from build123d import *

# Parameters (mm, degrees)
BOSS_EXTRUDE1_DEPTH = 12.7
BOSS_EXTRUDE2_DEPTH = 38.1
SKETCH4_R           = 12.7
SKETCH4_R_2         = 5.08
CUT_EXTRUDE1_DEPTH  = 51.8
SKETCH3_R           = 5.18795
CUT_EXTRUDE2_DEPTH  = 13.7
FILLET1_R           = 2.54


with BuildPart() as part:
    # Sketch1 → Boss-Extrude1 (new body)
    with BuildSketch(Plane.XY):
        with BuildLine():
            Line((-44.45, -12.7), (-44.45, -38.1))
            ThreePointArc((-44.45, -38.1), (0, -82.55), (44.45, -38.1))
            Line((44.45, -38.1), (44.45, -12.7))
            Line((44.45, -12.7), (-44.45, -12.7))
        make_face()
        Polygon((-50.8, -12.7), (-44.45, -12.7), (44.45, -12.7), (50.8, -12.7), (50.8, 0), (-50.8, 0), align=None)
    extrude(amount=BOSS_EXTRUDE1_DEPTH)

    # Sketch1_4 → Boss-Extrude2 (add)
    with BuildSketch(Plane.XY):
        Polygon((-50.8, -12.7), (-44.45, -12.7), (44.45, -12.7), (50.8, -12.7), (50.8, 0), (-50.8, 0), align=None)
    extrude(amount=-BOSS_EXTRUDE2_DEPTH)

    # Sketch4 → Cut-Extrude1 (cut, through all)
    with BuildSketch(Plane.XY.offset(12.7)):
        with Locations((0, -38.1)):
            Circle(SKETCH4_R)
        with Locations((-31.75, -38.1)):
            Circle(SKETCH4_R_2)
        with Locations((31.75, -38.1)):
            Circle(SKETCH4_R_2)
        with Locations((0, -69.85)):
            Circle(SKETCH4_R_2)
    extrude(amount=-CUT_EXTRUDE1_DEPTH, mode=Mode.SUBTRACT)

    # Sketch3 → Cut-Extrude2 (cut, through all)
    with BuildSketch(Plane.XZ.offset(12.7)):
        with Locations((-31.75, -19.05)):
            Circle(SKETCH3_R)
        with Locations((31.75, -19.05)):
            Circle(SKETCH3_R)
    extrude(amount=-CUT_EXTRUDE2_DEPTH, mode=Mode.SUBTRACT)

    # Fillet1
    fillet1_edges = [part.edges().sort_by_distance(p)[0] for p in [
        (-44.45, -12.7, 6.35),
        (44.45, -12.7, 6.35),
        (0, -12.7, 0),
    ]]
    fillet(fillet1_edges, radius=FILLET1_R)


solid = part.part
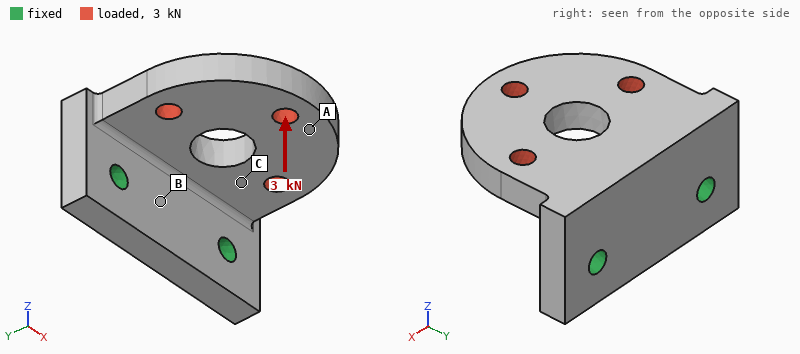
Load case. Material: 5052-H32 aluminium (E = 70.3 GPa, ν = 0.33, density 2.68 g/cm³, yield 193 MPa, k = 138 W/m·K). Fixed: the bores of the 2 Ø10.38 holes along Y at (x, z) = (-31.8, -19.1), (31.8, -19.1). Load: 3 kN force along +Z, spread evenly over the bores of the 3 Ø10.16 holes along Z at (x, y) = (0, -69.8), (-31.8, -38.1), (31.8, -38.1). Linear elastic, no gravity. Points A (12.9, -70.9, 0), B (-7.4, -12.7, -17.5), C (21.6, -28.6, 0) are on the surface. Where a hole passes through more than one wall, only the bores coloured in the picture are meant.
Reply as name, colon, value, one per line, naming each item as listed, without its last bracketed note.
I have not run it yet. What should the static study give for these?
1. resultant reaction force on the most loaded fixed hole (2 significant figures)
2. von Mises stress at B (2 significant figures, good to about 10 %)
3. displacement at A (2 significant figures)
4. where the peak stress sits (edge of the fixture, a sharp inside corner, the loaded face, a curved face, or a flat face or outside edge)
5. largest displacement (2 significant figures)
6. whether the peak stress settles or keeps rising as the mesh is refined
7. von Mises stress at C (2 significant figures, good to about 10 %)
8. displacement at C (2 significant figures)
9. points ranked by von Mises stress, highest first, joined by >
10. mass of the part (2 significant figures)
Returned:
resultant reaction force on the most loaded fixed hole: 1.5 kN
von Mises stress at B: 21 MPa
displacement at A: 0.30 mm
where the peak stress sits: edge of the fixture
largest displacement: 0.37 mm
whether the peak stress settles or keeps rising as the mesh is refined: keeps rising
von Mises stress at C: 37 MPa
displacement at C: 0.074 mm
points ranked by von Mises stress, highest first, joined by >: C > B > A
mass of the part: 330 g
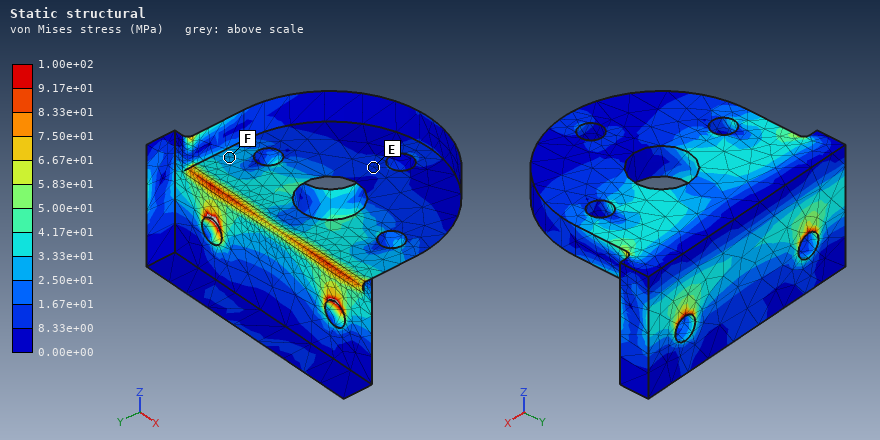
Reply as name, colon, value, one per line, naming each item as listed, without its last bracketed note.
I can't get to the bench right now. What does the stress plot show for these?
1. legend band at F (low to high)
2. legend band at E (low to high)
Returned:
legend band at F: 2.50e+01 to 3.33e+01 MPa
legend band at E: 8.33e+00 to 1.67e+01 MPa
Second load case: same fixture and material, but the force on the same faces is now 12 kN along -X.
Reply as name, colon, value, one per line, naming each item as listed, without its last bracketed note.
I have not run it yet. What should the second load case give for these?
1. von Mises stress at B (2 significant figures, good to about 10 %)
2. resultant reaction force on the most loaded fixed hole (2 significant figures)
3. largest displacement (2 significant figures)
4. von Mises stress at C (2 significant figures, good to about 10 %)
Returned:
von Mises stress at B: 28 MPa
resultant reaction force on the most loaded fixed hole: 10 kN
largest displacement: 0.18 mm
von Mises stress at C: 48 MPa
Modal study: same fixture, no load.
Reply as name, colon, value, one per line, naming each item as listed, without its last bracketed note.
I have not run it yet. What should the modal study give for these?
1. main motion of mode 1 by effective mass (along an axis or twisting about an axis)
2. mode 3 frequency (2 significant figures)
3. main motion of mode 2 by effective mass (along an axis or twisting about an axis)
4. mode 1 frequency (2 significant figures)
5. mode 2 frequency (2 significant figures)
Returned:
main motion of mode 1 by effective mass: along Z
mode 3 frequency: 5100 Hz
main motion of mode 2 by effective mass: along X
mode 1 frequency: 1500 Hz
mode 2 frequency: 3500 Hz
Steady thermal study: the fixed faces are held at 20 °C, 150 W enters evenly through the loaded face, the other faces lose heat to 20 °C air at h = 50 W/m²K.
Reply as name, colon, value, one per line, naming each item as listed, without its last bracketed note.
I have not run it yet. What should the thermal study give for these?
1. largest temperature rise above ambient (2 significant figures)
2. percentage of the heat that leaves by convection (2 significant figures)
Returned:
largest temperature rise above ambient: 66 K
percentage of the heat that leaves by convection: 22 %
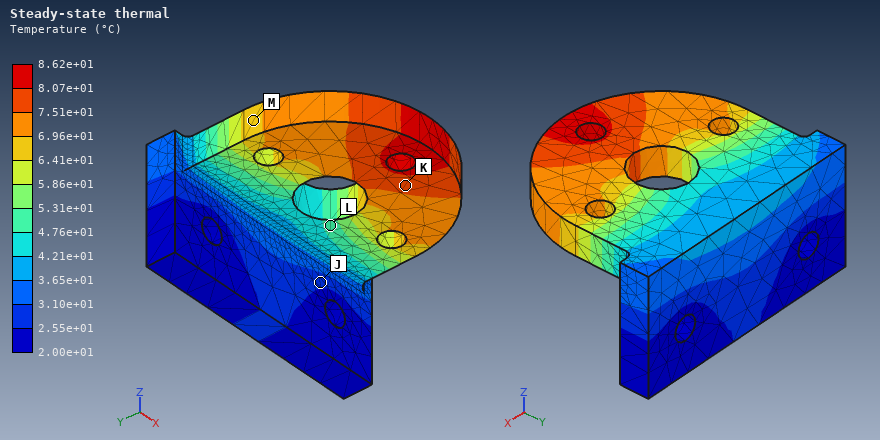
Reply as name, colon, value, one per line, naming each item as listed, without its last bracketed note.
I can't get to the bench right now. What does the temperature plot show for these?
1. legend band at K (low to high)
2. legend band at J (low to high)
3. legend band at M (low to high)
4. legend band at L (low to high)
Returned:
legend band at K: 7.51e+01 to 8.07e+01 °C
legend band at J: 2.55e+01 to 3.10e+01 °C
legend band at M: 6.41e+01 to 6.96e+01 °C
legend band at L: 4.76e+01 to 5.31e+01 °C
